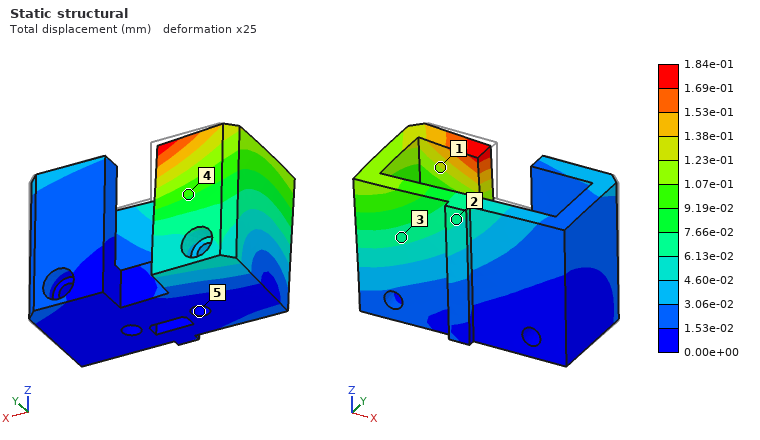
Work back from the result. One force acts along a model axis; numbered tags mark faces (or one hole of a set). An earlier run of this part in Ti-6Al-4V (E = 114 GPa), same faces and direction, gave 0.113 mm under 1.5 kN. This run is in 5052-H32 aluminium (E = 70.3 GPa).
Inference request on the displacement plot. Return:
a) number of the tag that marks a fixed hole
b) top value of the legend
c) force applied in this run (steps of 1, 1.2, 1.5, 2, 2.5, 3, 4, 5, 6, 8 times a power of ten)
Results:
5
1.84e-01 mm
1.5 kN
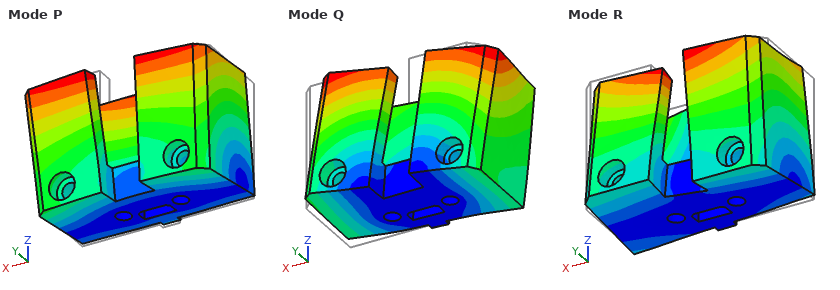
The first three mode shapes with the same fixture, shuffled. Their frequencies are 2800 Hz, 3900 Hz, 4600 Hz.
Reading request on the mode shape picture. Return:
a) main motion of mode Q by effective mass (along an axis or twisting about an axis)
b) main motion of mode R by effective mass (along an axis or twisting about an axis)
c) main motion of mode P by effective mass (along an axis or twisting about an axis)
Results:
along X
twisting about Z
along Y
